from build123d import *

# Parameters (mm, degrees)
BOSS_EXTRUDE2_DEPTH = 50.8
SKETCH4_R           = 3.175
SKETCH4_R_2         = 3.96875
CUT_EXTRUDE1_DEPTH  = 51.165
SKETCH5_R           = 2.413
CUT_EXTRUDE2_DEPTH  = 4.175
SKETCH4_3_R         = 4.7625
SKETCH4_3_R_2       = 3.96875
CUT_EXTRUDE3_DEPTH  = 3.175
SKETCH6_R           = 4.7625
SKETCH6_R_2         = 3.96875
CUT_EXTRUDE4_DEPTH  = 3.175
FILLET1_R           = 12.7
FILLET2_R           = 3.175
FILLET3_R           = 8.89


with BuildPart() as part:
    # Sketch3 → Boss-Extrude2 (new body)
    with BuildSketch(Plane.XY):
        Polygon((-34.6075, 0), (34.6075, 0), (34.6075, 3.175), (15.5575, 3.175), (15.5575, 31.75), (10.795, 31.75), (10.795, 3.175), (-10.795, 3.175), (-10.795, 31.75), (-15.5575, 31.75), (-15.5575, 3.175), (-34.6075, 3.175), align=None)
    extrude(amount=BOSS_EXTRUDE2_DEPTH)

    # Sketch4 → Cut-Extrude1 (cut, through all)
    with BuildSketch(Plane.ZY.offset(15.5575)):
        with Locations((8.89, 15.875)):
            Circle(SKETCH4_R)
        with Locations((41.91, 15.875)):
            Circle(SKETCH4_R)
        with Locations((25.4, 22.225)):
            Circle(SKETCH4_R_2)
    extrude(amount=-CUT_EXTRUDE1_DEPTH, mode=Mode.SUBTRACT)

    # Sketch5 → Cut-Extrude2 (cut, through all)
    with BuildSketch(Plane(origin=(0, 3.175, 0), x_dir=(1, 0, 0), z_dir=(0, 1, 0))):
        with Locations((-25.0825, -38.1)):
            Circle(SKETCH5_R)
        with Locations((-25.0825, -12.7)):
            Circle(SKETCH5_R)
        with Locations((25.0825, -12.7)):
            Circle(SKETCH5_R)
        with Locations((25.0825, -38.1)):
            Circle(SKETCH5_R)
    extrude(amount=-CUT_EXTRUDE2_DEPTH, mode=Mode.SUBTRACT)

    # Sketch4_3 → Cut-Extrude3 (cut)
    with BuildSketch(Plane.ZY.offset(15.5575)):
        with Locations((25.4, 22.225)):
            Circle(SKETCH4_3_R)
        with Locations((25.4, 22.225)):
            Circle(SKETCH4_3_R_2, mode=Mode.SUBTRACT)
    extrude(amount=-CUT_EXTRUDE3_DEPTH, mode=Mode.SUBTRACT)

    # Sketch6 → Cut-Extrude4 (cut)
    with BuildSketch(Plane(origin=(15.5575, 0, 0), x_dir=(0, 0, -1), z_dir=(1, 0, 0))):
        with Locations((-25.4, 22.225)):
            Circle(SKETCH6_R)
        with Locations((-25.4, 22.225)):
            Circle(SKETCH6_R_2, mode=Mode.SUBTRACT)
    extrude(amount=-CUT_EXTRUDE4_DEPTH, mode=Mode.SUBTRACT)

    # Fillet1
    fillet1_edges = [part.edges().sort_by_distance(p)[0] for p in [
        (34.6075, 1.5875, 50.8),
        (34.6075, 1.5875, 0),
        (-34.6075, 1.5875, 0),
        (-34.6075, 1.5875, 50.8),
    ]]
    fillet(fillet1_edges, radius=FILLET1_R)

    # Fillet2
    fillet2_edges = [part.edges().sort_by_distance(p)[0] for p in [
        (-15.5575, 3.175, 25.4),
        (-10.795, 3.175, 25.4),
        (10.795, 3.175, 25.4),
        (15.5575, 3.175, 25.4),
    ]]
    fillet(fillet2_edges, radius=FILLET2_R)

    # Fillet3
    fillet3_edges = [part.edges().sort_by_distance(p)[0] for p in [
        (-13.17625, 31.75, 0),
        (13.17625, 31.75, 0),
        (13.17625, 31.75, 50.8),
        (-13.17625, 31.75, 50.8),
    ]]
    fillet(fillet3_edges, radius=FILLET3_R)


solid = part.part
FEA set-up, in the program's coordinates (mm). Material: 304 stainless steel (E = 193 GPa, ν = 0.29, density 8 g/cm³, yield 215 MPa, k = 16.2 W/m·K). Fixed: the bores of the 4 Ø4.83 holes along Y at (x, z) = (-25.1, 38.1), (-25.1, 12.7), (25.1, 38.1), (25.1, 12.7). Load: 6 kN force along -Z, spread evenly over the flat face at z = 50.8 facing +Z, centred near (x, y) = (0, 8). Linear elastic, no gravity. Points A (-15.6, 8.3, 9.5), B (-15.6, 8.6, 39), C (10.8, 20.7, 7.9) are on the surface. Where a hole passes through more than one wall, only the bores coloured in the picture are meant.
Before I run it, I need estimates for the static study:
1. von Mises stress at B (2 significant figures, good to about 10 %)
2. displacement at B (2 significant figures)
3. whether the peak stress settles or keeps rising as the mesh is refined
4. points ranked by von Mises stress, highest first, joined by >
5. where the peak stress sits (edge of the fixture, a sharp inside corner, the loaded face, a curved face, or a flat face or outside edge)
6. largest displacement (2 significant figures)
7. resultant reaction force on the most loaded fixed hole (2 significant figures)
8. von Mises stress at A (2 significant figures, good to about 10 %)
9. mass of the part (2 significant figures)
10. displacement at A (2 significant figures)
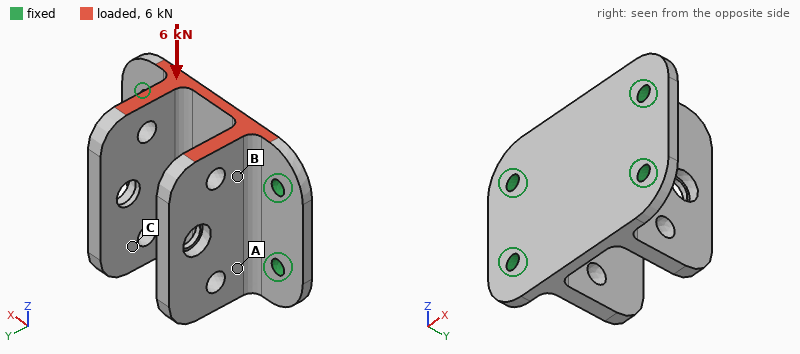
42 MPa
12 µm
keeps rising
B > A > C
edge of the fixture
30 µm
1.9 kN
26 MPa
190 g
12 µm
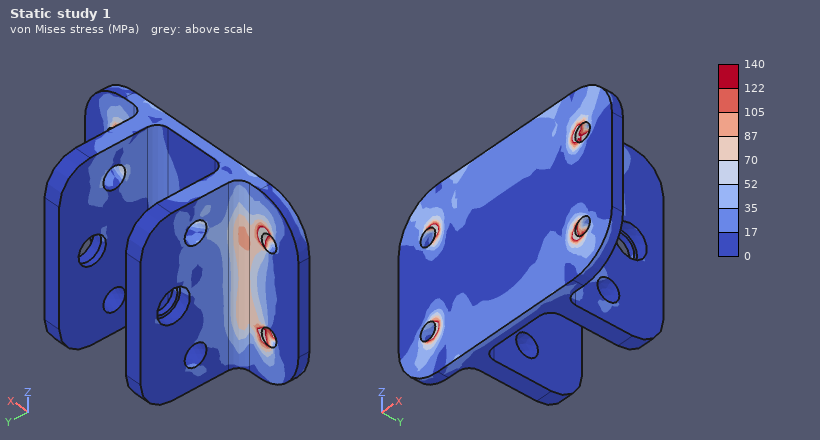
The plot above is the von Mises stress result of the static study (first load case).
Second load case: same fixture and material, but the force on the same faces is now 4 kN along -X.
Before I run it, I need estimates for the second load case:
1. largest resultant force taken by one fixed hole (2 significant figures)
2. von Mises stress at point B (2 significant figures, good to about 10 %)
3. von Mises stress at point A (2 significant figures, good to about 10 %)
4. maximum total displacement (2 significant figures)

2.0 kN
64 MPa
14 MPa
65 µm
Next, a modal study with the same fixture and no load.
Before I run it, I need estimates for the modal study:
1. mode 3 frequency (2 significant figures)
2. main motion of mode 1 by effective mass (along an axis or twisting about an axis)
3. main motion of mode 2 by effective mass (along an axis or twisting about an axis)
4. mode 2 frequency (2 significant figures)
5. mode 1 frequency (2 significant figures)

4200 Hz
along Y
along X
4000 Hz
2400 Hz
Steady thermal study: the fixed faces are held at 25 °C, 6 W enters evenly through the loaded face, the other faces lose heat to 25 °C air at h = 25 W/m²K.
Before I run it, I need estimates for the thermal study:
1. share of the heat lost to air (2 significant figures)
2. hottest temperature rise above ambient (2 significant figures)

40 %
24 K
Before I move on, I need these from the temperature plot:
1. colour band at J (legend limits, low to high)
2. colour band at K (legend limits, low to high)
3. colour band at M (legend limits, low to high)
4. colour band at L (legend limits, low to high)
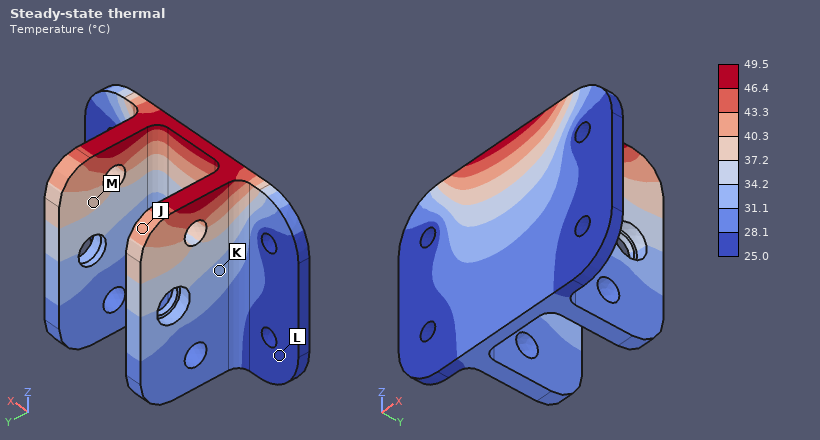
40.3 to 43.3 °C
31.1 to 34.2 °C
37.2 to 40.3 °C
25.0 to 28.1 °C
